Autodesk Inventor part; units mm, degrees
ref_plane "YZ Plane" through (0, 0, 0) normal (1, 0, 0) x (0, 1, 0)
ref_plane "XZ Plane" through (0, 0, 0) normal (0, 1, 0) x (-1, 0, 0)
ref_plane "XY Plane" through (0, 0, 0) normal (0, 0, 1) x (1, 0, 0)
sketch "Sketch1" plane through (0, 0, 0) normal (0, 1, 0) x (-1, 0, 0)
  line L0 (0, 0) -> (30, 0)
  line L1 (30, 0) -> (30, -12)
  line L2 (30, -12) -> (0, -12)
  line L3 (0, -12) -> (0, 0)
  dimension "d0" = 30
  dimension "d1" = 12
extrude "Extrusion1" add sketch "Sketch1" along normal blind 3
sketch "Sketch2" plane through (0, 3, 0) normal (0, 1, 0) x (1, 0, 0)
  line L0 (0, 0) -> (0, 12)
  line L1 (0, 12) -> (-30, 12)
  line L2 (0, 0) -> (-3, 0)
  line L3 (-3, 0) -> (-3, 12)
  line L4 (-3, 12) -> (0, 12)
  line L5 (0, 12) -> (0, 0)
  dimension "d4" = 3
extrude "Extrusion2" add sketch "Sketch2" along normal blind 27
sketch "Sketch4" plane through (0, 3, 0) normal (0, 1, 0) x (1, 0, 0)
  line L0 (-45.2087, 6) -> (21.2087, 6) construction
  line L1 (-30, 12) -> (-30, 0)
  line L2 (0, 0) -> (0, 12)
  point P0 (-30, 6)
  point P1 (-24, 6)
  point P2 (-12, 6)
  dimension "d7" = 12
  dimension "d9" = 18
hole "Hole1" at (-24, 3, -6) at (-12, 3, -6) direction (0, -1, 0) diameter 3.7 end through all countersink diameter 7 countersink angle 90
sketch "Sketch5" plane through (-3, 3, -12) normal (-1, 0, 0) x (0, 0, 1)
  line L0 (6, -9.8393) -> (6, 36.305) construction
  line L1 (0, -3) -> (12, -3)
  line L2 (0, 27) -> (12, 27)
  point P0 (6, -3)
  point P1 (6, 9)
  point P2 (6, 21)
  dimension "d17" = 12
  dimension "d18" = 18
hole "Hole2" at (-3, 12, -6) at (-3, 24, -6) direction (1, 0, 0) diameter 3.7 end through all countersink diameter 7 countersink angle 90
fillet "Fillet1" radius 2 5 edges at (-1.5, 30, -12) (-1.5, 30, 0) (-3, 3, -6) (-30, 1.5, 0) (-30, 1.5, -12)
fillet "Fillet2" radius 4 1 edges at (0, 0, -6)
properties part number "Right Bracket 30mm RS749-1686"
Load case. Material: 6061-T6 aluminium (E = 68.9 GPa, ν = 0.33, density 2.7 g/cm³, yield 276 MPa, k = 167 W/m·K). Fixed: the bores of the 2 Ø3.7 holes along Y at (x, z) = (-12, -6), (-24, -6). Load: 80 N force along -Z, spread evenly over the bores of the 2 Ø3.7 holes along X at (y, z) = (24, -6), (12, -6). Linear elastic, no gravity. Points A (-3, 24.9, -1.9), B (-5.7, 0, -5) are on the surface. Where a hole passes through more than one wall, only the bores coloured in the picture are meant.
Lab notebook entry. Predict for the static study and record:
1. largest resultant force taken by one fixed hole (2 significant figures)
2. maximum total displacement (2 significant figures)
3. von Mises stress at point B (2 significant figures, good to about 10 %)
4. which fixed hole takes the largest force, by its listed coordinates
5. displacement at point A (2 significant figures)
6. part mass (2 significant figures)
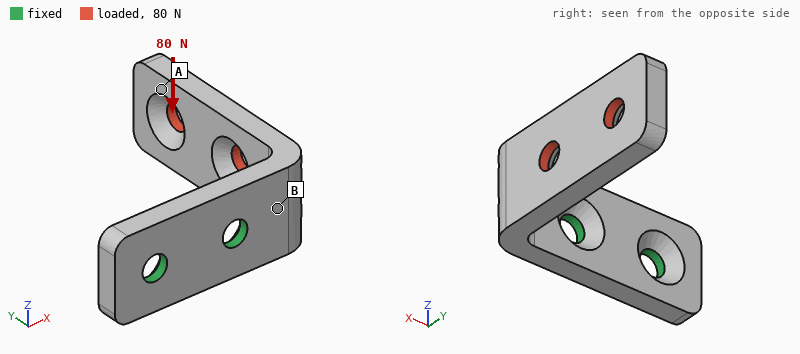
100 N
0.18 mm
54 MPa
(-12, -6)
0.15 mm
4.9 g
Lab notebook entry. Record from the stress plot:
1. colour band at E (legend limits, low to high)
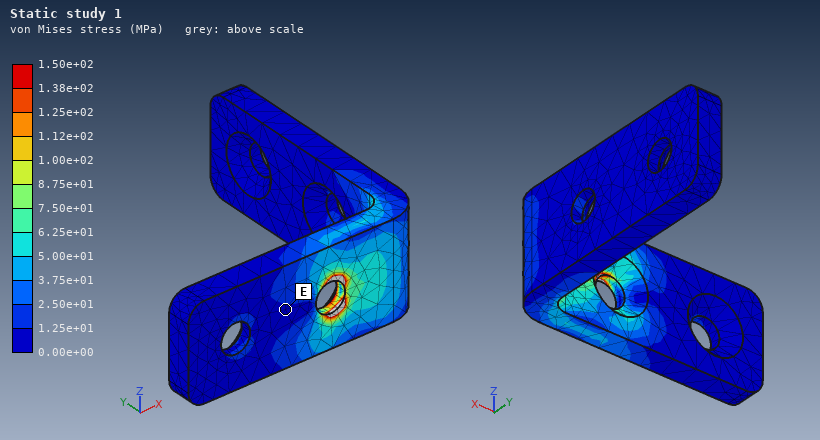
0.00e+00 to 1.25e+01 MPa
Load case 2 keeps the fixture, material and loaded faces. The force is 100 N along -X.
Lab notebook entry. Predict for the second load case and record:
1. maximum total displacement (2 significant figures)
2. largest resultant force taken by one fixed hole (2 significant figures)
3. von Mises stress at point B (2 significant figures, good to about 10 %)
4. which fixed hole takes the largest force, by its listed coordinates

0.47 mm
180 N
79 MPa
(-24, -6)
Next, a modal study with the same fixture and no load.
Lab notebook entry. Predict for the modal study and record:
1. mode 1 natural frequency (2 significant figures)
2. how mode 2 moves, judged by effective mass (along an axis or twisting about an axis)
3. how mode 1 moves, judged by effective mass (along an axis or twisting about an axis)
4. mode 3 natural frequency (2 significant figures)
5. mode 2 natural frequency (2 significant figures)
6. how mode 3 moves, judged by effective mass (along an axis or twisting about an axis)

1900 Hz
along Z
along X
7600 Hz
2800 Hz
along Y
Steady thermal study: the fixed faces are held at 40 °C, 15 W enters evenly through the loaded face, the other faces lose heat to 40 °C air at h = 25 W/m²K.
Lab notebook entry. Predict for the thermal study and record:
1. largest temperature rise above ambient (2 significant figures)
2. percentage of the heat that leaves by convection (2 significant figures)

70 K
8.0 %
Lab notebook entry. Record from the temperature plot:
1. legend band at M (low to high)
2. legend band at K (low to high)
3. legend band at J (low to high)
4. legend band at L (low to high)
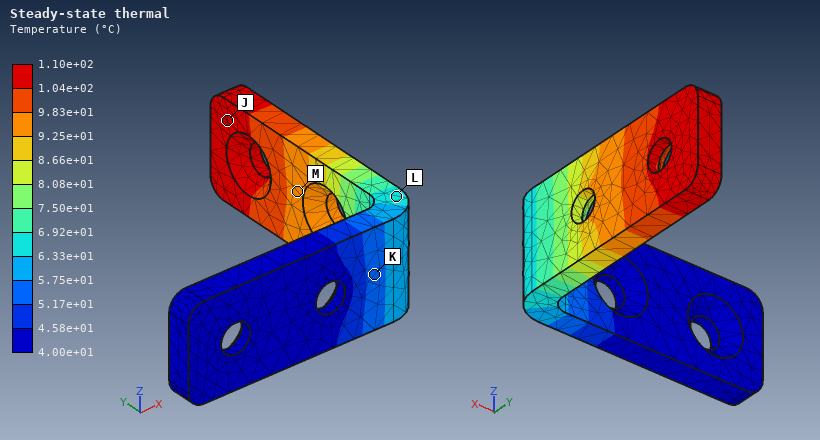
9.25e+01 to 9.83e+01 °C
5.17e+01 to 5.75e+01 °C
1.04e+02 to 1.10e+02 °C
6.33e+01 to 6.92e+01 °C
